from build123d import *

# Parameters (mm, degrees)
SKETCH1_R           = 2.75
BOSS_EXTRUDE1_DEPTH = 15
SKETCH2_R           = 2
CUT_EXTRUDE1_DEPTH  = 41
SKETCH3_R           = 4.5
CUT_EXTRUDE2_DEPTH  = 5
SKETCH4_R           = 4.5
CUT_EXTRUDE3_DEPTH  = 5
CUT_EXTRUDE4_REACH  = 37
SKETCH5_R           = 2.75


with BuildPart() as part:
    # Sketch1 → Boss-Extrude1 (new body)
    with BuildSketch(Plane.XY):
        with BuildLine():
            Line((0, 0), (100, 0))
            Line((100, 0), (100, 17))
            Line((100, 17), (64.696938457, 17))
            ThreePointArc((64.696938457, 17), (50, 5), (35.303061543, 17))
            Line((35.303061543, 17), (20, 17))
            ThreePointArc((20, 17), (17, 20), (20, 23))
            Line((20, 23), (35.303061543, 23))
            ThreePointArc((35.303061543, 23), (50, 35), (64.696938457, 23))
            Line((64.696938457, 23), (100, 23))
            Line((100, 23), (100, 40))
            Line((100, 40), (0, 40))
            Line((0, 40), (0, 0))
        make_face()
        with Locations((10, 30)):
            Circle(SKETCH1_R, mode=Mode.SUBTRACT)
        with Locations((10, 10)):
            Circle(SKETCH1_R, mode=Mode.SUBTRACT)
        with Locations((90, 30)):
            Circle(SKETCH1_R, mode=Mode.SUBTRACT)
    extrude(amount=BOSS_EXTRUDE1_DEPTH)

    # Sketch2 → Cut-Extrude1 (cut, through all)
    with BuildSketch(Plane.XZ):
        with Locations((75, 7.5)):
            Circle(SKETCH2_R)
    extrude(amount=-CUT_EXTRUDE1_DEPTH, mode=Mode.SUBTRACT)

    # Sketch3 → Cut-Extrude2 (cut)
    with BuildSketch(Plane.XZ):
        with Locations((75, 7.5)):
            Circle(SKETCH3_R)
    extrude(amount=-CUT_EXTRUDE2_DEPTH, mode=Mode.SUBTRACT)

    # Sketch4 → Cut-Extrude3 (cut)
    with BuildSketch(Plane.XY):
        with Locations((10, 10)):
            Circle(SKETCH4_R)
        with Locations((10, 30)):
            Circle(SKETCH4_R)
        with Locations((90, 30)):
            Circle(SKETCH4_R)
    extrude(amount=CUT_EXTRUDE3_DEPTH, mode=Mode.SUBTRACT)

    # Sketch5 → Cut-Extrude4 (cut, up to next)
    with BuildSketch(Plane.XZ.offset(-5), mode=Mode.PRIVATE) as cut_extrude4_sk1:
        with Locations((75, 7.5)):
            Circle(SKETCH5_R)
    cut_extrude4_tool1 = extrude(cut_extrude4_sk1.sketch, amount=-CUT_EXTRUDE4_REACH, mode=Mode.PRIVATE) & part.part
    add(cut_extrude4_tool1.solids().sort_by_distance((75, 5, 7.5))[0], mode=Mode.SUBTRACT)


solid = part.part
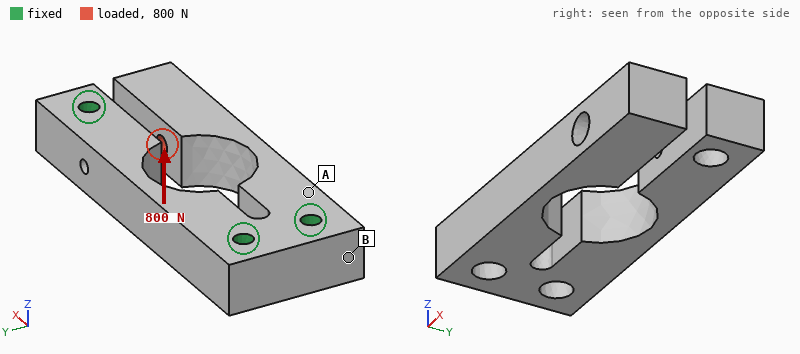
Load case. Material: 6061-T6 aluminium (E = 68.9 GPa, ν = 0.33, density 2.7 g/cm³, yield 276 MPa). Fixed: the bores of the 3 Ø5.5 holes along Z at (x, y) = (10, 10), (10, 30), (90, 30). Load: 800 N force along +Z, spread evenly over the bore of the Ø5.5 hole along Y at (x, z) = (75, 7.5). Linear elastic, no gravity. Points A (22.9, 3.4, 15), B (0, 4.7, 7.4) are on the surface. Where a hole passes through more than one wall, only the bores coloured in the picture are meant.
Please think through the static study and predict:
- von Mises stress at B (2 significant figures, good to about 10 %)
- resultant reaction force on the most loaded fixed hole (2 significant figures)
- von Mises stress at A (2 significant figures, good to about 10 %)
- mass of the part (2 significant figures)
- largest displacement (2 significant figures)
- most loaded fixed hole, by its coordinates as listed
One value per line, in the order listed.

22 MPa
860 N
68 MPa
110 g
0.73 mm
(10, 10)
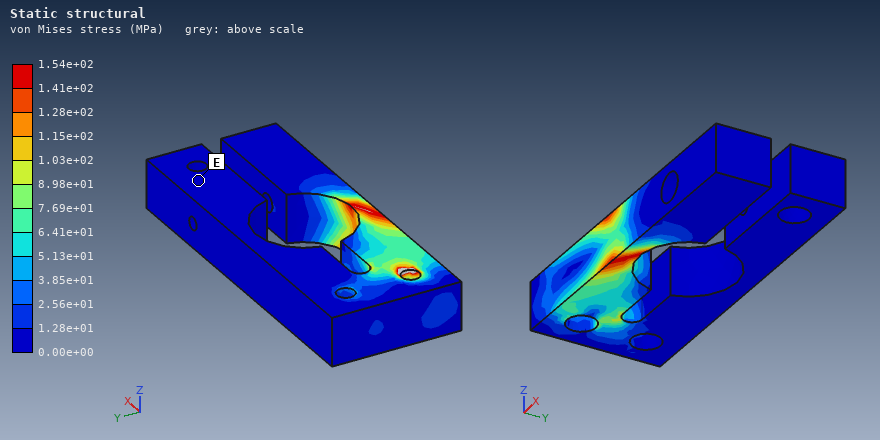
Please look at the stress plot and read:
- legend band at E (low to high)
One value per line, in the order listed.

0.00e+00 to 1.28e+01 MPa
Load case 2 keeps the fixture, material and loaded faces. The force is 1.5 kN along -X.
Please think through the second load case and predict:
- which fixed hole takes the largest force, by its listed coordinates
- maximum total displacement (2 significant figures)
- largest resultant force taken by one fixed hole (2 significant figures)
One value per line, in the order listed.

(10, 10)
0.86 mm
1.4 kN
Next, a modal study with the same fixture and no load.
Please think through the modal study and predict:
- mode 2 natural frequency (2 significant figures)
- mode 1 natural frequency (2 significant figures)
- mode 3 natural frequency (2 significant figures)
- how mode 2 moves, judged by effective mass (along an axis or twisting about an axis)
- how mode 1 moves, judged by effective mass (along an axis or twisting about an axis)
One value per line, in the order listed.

1200 Hz
730 Hz
4500 Hz
along Z
along Y
